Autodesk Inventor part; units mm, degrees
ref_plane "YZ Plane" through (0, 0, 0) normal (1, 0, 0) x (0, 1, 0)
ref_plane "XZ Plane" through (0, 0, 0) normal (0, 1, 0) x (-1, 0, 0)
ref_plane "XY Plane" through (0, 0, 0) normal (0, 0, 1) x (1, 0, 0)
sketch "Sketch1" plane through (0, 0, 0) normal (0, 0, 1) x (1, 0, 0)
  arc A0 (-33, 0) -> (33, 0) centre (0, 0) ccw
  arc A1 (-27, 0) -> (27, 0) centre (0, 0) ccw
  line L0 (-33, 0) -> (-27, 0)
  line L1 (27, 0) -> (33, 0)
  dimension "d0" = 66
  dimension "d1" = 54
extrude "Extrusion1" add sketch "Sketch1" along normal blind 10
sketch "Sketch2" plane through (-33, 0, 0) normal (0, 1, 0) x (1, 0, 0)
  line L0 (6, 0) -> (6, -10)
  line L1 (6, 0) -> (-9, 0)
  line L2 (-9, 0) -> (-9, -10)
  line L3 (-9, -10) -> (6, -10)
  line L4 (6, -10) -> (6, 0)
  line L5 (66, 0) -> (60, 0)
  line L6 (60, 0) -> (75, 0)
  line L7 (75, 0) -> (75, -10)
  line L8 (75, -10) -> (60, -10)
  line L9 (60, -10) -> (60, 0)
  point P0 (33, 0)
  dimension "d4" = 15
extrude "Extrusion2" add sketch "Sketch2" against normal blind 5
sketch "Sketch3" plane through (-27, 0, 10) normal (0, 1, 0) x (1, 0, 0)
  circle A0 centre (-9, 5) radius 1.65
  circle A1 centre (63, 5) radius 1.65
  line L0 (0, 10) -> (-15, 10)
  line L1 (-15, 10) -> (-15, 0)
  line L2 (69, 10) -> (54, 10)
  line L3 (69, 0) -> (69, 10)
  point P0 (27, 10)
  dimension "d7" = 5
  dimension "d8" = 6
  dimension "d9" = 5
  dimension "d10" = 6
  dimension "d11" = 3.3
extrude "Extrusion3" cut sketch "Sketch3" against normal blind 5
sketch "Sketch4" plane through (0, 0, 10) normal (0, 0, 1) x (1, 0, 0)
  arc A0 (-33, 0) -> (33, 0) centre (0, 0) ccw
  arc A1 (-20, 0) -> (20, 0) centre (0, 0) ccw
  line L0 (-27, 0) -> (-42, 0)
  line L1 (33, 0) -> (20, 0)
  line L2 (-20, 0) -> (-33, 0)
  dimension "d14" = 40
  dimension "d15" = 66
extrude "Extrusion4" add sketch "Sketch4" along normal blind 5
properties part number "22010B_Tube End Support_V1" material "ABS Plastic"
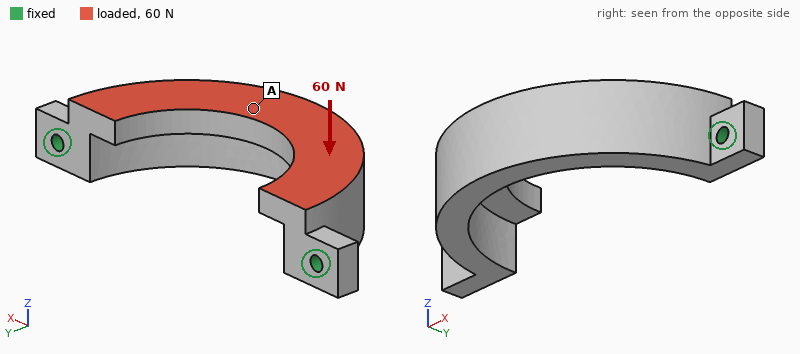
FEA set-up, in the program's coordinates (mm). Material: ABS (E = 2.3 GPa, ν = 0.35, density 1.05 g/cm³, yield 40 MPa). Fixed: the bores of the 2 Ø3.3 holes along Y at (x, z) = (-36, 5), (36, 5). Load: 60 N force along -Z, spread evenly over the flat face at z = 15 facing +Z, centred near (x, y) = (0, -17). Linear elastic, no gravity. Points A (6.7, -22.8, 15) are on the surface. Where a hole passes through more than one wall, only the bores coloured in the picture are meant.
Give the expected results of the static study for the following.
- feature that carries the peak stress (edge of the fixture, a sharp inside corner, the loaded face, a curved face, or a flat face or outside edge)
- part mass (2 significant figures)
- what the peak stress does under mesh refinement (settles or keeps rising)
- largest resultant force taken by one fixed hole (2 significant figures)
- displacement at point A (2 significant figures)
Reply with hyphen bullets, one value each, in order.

- edge of the fixture
- 12 g
- keeps rising
- 31 N
- 0.22 mm
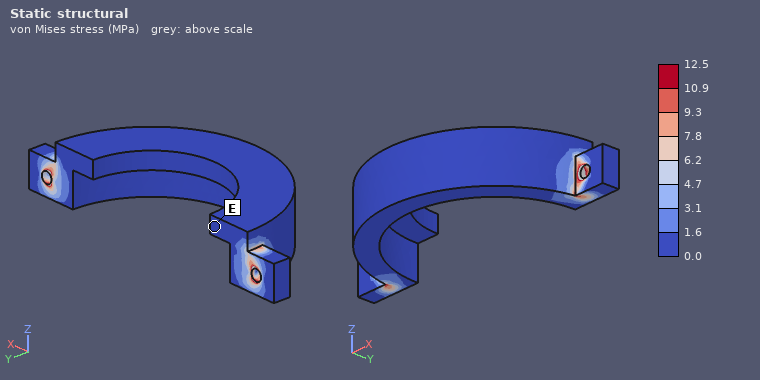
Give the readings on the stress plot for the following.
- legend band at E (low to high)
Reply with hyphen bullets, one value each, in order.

- 0.0 to 1.6 MPa
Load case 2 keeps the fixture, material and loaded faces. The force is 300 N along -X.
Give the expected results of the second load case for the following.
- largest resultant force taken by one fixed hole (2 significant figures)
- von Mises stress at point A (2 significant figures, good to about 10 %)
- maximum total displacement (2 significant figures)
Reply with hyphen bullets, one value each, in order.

- 160 N
- 4.3 MPa
- 0.15 mm
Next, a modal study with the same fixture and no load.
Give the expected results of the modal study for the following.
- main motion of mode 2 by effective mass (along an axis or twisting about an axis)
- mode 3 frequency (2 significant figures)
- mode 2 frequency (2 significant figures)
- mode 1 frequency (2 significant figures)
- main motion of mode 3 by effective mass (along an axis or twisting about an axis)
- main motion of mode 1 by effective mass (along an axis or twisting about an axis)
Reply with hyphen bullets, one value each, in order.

- along X
- 3000 Hz
- 2200 Hz
- 760 Hz
- along X
- along Z
